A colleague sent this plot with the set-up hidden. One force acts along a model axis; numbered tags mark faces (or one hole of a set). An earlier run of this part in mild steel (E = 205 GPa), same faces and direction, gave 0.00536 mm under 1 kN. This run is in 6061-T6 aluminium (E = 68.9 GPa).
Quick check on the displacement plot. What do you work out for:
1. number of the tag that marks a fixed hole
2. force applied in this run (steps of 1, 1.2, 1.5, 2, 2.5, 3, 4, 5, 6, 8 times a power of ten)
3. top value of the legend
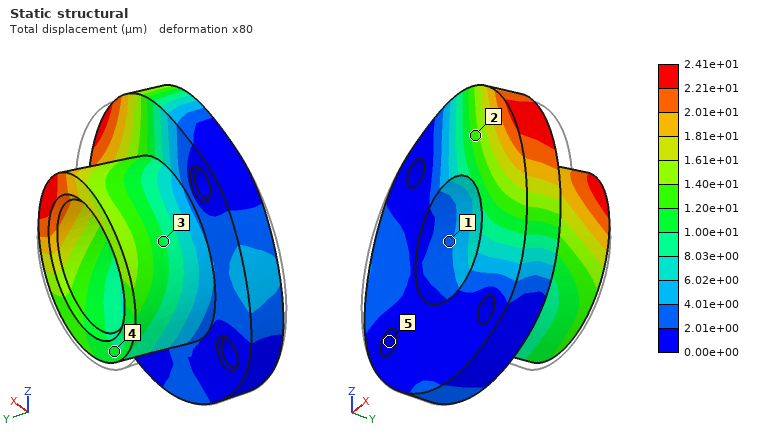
5
1.5 kN
2.41e+01 µm
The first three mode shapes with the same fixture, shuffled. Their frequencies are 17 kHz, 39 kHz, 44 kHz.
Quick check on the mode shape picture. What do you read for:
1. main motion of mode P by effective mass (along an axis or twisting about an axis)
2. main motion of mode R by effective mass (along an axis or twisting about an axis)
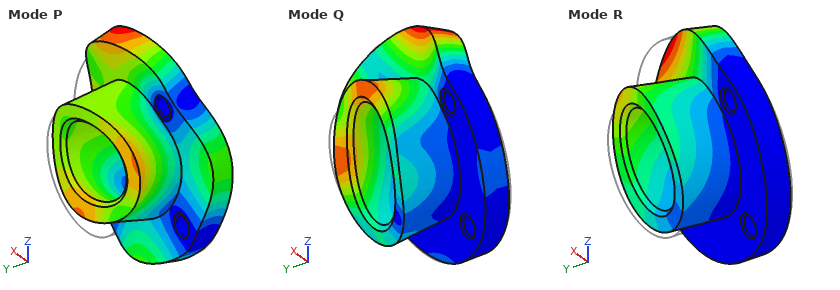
along Z
along Y
